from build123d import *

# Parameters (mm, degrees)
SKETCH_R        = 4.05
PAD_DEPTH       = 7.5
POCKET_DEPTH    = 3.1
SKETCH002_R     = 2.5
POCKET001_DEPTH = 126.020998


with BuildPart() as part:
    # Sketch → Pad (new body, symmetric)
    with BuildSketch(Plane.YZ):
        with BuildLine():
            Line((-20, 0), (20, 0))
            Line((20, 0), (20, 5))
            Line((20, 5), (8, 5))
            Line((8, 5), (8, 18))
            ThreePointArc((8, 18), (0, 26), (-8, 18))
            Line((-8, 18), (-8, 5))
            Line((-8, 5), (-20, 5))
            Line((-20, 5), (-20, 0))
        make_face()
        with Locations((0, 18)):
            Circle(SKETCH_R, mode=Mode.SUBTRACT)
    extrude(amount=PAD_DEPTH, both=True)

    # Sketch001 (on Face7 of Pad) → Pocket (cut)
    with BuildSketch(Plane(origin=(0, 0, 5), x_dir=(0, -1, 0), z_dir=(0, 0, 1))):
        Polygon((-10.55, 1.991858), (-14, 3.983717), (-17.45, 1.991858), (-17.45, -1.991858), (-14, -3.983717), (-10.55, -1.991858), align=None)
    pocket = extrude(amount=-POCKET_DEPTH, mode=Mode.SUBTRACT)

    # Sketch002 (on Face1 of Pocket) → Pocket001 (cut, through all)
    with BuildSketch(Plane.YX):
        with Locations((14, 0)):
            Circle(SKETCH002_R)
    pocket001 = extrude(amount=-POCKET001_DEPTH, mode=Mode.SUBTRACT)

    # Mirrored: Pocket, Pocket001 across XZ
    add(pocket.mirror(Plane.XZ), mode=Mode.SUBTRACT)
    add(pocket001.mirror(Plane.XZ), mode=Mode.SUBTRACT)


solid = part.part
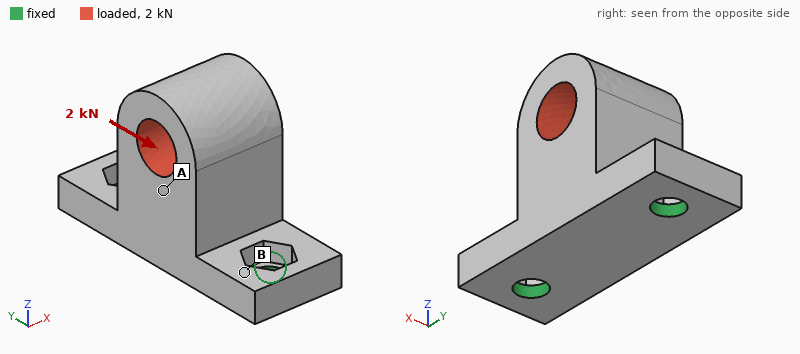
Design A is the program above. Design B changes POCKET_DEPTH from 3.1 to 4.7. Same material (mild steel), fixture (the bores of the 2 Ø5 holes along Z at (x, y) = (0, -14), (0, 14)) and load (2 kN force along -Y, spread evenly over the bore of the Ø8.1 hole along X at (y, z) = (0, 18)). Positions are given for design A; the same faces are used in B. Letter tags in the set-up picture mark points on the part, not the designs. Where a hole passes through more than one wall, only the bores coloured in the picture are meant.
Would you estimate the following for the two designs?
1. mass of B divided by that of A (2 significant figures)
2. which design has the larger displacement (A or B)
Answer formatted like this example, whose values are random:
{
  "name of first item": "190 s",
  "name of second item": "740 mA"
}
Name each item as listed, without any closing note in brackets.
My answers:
{
  "mass of B divided by that of A": "0.99",
  "which design has the larger displacement": "B"
}
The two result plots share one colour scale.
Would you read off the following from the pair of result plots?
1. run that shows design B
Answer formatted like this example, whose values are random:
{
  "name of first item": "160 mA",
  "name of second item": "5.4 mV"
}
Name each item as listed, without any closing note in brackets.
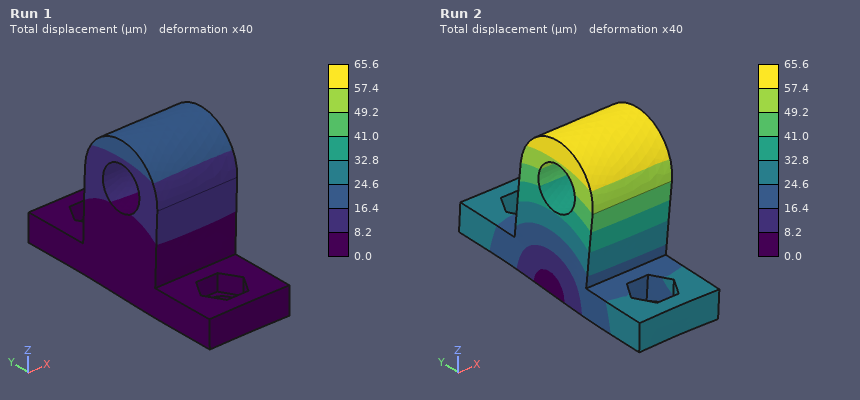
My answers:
{
  "run that shows design B": "Run 2"
}
